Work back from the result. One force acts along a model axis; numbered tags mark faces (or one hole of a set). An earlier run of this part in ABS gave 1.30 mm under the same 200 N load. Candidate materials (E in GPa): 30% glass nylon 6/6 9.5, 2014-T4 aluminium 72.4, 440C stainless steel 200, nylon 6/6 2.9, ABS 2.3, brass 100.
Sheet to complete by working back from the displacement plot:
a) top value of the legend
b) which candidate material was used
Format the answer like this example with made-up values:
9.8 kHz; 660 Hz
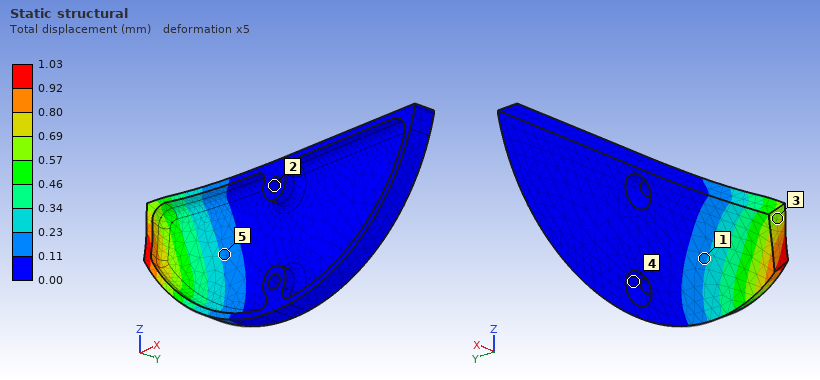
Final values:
1.03 mm; nylon 6/6
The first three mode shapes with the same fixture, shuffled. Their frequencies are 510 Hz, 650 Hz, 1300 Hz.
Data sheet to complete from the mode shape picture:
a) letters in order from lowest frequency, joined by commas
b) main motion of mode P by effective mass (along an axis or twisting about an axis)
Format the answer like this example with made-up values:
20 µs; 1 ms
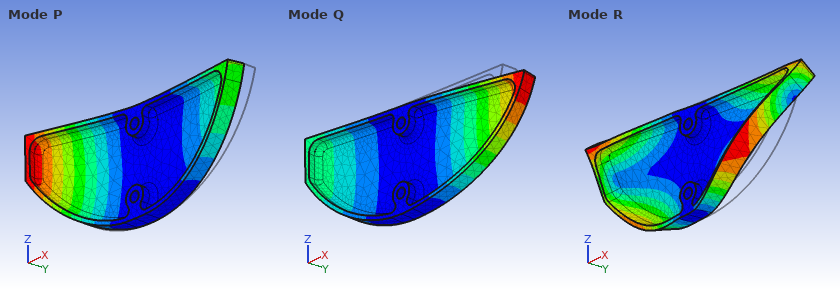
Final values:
Q, P, R; along Y
